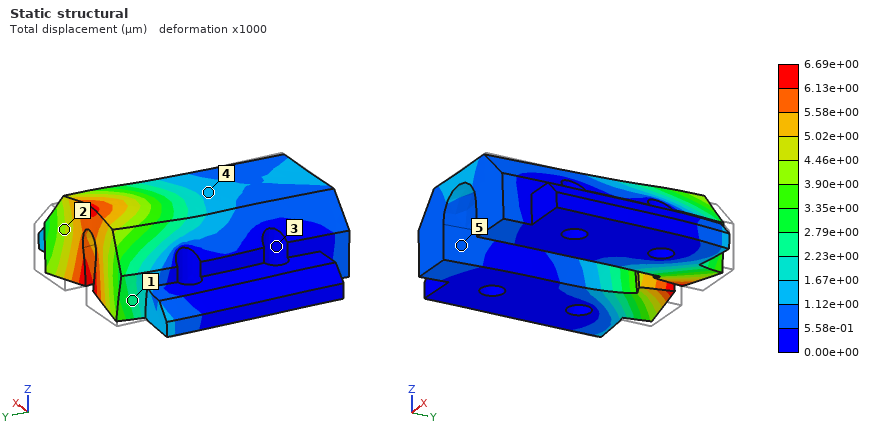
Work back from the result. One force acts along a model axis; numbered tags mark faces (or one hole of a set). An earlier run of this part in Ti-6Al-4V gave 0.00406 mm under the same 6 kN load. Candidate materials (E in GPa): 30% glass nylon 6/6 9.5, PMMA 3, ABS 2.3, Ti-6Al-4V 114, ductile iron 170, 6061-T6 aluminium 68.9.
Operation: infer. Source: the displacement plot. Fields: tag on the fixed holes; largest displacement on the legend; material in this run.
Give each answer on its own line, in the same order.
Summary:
3
6.69e+00 µm
6061-T6 aluminium
